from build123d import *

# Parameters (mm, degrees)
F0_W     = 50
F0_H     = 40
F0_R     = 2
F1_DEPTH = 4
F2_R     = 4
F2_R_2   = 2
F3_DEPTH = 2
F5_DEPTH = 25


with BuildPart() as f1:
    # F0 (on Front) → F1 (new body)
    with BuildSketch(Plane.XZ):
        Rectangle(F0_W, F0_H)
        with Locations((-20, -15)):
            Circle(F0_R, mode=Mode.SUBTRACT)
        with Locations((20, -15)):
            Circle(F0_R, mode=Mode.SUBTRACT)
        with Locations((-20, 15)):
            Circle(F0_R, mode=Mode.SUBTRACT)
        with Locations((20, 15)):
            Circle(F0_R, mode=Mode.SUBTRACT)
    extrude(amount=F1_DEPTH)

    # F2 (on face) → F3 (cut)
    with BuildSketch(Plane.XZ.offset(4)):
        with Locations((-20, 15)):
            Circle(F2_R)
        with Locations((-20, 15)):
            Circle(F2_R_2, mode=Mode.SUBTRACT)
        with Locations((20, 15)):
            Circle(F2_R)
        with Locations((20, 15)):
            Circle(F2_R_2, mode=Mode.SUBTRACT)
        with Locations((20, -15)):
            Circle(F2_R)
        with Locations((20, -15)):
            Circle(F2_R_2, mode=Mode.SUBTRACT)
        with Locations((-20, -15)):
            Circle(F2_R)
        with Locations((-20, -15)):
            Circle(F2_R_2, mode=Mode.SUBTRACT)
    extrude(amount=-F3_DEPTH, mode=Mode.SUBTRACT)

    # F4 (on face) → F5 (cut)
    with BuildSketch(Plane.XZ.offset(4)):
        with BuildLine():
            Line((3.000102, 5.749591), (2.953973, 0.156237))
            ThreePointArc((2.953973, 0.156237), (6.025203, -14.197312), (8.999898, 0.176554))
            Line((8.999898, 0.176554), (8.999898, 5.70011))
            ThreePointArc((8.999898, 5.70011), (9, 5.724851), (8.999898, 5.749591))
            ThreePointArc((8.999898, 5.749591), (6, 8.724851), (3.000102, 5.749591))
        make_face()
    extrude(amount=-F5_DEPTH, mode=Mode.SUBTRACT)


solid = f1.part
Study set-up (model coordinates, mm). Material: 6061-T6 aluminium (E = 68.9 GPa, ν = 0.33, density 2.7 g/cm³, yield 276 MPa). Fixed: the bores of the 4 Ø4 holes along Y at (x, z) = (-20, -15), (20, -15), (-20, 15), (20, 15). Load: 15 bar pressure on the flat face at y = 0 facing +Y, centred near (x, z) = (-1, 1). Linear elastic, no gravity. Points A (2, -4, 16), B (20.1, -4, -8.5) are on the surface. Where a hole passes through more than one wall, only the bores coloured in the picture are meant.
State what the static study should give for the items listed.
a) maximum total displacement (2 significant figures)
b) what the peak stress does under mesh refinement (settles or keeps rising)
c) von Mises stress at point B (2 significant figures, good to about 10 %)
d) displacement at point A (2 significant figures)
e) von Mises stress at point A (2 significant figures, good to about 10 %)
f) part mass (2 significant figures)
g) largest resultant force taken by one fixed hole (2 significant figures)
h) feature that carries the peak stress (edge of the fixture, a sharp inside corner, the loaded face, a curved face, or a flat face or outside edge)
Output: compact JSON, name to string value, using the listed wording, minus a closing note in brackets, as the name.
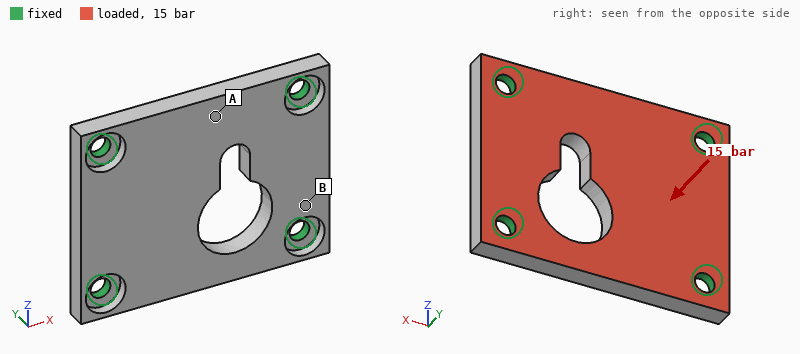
{"maximum total displacement": "85 µm", "what the peak stress does under mesh refinement": "keeps rising", "von Mises stress at point B": "35 MPa", "displacement at point A": "52 µm", "von Mises stress at point A": "68 MPa", "part mass": "18 g", "largest resultant force taken by one fixed hole": "860 N", "feature that carries the peak stress": "edge of the fixture"}
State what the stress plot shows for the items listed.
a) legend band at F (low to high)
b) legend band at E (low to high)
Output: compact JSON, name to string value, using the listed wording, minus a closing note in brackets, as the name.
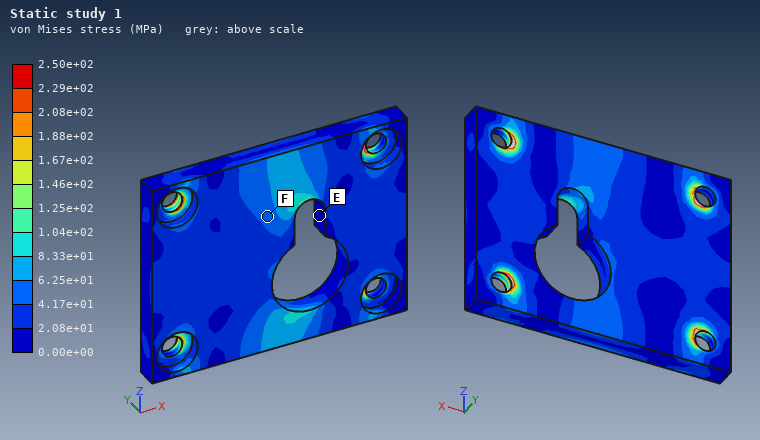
{"legend band at F": "4.17e+01 to 6.25e+01 MPa", "legend band at E": "0.00e+00 to 2.08e+01 MPa"}
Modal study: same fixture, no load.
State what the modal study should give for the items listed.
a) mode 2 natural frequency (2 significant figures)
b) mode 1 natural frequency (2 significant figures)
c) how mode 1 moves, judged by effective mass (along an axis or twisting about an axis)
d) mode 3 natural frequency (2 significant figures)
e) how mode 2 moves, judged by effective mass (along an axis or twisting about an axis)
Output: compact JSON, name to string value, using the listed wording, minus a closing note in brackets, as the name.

{"mode 2 natural frequency": "12 kHz", "mode 1 natural frequency": "8500 Hz", "how mode 1 moves, judged by effective mass": "along Y", "mode 3 natural frequency": "16 kHz", "how mode 2 moves, judged by effective mass": "twisting about X"}
